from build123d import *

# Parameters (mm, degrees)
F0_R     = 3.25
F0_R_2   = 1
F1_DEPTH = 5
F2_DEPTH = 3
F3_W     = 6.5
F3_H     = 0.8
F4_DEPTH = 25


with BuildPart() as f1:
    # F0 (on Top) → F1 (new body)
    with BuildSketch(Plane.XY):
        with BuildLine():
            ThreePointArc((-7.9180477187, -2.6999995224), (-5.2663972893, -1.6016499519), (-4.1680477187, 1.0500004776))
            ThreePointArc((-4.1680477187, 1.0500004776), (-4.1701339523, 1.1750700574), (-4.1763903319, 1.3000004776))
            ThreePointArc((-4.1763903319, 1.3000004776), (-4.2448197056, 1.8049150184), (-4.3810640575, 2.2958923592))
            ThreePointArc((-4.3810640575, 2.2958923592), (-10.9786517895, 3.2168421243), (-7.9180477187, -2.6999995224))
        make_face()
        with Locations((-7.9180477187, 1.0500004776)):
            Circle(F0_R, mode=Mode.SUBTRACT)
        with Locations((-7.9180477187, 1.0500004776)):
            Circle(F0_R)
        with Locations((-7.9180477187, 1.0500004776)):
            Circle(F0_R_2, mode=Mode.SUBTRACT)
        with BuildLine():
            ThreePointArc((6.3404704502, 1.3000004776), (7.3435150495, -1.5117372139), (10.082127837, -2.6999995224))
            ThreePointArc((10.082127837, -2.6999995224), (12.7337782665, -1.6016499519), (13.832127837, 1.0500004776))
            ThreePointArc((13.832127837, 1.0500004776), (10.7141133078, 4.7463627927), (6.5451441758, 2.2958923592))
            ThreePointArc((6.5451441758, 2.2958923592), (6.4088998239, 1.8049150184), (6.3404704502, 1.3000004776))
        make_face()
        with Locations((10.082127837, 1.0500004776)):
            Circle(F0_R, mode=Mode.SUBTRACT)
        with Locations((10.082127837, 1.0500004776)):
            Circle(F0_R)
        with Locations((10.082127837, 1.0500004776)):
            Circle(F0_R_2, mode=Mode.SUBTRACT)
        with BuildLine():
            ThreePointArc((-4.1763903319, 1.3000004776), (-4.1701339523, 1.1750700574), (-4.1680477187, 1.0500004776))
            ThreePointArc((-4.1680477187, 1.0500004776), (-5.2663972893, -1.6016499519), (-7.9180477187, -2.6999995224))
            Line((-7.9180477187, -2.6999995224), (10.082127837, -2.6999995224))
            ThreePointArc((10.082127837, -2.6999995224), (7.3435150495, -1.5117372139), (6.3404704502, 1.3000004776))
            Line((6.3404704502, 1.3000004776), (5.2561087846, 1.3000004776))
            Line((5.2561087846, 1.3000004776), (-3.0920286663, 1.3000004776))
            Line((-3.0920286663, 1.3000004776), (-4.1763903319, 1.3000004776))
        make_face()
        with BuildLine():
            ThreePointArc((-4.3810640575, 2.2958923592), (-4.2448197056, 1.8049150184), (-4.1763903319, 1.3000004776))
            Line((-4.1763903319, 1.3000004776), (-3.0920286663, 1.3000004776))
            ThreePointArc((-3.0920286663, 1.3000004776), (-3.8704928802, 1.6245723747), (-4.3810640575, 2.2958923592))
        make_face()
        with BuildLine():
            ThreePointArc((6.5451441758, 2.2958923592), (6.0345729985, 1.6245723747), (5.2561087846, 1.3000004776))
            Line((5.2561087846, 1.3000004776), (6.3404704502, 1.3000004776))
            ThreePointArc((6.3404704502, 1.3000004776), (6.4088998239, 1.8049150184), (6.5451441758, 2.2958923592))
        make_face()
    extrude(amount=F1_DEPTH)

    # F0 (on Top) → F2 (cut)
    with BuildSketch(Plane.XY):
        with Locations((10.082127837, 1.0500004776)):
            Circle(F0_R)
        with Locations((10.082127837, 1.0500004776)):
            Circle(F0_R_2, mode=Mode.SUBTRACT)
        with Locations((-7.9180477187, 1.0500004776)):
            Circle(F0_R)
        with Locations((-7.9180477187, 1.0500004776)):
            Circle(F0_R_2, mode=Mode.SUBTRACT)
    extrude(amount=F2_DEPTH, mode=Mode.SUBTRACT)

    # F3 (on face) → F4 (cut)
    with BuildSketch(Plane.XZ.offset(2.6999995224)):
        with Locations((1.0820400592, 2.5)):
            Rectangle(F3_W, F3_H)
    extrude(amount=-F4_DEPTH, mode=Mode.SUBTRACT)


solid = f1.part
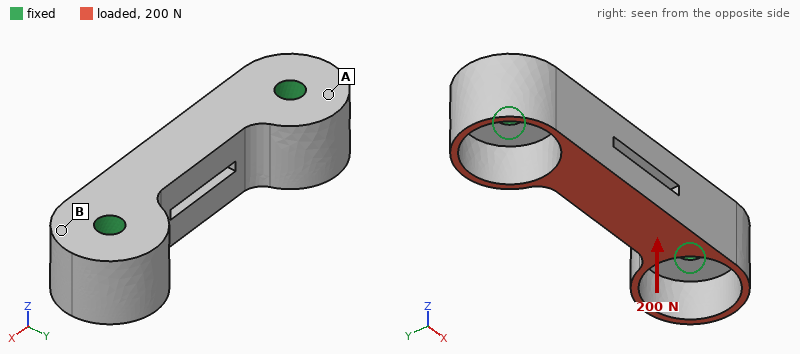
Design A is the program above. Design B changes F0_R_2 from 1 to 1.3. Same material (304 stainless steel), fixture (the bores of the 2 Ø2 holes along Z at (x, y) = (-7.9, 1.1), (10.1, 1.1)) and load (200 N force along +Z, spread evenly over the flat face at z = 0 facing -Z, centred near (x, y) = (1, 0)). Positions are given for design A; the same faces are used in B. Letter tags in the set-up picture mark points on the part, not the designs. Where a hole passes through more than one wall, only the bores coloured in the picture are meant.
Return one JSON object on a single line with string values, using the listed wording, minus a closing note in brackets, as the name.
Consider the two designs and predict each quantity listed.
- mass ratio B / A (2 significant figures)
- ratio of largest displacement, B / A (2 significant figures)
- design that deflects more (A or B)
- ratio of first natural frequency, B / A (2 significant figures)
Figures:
{"mass ratio B / A": "0.98", "ratio of largest displacement, B / A": "0.84", "design that deflects more": "A", "ratio of first natural frequency, B / A": "1.1"}
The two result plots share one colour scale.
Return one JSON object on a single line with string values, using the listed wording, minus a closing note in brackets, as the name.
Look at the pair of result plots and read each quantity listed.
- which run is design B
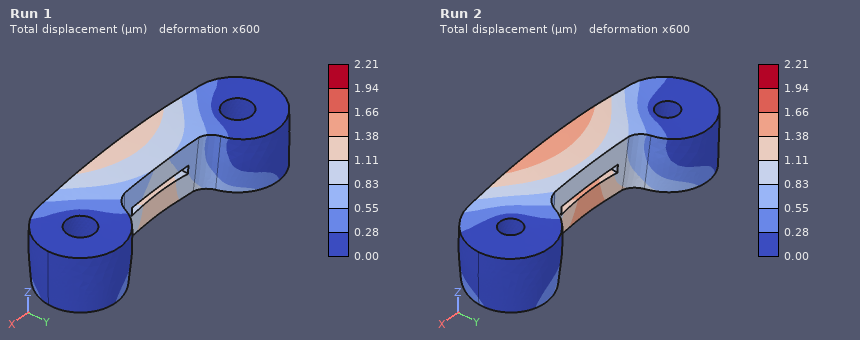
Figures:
{"which run is design B": "Run 1"}
